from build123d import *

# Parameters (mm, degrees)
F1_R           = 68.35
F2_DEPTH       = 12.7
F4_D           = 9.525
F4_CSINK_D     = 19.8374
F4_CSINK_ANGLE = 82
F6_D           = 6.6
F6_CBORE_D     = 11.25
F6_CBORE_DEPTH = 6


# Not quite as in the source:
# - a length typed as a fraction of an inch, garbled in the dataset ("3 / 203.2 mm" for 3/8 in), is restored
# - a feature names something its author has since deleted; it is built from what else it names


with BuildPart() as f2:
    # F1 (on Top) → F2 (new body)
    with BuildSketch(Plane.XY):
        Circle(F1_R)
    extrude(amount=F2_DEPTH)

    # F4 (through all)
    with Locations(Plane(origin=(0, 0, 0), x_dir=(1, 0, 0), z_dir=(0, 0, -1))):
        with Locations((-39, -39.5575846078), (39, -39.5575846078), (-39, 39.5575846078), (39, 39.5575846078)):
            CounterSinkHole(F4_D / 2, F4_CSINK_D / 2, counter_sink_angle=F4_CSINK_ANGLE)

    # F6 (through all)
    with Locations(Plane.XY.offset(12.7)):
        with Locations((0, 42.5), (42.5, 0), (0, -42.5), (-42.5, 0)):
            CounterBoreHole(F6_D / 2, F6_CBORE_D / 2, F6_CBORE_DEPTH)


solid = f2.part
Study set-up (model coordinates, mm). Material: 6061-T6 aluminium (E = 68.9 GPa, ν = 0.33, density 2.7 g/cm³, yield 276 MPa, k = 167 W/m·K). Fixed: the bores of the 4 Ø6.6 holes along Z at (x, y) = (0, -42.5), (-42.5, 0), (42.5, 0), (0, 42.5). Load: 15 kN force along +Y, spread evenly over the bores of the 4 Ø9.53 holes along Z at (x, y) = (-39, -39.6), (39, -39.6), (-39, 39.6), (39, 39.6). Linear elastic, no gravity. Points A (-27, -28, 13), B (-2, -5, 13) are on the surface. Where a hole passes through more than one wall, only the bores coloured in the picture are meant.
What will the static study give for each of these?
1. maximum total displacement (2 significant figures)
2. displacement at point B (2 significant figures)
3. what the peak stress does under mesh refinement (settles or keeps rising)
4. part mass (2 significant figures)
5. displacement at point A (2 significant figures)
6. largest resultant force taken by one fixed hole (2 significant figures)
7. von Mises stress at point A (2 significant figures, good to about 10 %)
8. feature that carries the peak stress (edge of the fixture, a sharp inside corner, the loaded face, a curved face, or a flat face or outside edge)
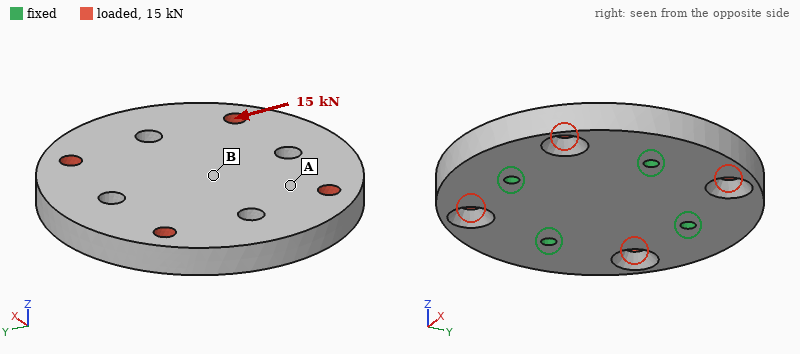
18 µm
3.5 µm
keeps rising
480 g
6.7 µm
4.6 kN
11 MPa
edge of the fixture
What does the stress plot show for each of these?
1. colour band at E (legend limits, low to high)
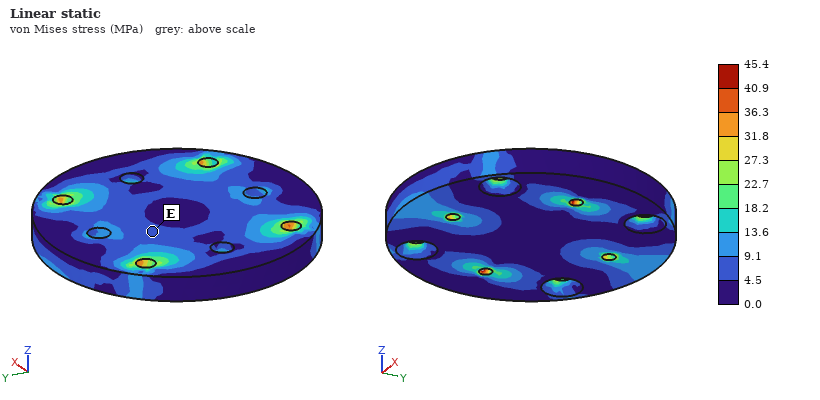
4.5 to 9.1 MPa
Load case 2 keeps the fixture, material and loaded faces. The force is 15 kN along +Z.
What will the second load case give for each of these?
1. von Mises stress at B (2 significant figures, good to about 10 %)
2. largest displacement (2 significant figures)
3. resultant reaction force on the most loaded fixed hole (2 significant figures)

16 MPa
76 µm
3.9 kN
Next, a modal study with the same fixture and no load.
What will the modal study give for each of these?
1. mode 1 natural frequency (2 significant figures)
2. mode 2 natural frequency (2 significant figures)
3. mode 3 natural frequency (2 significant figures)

4700 Hz
5700 Hz
5800 Hz
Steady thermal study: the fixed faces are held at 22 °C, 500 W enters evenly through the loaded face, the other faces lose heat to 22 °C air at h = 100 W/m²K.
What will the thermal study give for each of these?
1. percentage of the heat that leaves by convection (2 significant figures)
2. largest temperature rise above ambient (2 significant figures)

17 %
55 K
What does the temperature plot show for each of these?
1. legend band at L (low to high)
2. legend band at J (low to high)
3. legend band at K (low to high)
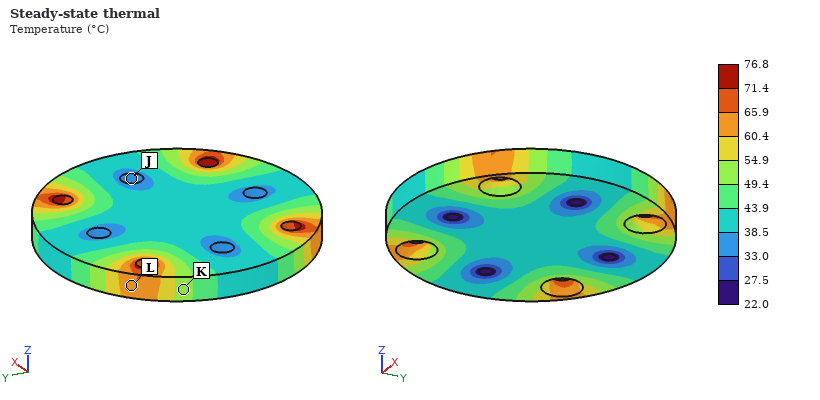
60.4 to 65.9 °C
33.0 to 38.5 °C
49.4 to 54.9 °C
